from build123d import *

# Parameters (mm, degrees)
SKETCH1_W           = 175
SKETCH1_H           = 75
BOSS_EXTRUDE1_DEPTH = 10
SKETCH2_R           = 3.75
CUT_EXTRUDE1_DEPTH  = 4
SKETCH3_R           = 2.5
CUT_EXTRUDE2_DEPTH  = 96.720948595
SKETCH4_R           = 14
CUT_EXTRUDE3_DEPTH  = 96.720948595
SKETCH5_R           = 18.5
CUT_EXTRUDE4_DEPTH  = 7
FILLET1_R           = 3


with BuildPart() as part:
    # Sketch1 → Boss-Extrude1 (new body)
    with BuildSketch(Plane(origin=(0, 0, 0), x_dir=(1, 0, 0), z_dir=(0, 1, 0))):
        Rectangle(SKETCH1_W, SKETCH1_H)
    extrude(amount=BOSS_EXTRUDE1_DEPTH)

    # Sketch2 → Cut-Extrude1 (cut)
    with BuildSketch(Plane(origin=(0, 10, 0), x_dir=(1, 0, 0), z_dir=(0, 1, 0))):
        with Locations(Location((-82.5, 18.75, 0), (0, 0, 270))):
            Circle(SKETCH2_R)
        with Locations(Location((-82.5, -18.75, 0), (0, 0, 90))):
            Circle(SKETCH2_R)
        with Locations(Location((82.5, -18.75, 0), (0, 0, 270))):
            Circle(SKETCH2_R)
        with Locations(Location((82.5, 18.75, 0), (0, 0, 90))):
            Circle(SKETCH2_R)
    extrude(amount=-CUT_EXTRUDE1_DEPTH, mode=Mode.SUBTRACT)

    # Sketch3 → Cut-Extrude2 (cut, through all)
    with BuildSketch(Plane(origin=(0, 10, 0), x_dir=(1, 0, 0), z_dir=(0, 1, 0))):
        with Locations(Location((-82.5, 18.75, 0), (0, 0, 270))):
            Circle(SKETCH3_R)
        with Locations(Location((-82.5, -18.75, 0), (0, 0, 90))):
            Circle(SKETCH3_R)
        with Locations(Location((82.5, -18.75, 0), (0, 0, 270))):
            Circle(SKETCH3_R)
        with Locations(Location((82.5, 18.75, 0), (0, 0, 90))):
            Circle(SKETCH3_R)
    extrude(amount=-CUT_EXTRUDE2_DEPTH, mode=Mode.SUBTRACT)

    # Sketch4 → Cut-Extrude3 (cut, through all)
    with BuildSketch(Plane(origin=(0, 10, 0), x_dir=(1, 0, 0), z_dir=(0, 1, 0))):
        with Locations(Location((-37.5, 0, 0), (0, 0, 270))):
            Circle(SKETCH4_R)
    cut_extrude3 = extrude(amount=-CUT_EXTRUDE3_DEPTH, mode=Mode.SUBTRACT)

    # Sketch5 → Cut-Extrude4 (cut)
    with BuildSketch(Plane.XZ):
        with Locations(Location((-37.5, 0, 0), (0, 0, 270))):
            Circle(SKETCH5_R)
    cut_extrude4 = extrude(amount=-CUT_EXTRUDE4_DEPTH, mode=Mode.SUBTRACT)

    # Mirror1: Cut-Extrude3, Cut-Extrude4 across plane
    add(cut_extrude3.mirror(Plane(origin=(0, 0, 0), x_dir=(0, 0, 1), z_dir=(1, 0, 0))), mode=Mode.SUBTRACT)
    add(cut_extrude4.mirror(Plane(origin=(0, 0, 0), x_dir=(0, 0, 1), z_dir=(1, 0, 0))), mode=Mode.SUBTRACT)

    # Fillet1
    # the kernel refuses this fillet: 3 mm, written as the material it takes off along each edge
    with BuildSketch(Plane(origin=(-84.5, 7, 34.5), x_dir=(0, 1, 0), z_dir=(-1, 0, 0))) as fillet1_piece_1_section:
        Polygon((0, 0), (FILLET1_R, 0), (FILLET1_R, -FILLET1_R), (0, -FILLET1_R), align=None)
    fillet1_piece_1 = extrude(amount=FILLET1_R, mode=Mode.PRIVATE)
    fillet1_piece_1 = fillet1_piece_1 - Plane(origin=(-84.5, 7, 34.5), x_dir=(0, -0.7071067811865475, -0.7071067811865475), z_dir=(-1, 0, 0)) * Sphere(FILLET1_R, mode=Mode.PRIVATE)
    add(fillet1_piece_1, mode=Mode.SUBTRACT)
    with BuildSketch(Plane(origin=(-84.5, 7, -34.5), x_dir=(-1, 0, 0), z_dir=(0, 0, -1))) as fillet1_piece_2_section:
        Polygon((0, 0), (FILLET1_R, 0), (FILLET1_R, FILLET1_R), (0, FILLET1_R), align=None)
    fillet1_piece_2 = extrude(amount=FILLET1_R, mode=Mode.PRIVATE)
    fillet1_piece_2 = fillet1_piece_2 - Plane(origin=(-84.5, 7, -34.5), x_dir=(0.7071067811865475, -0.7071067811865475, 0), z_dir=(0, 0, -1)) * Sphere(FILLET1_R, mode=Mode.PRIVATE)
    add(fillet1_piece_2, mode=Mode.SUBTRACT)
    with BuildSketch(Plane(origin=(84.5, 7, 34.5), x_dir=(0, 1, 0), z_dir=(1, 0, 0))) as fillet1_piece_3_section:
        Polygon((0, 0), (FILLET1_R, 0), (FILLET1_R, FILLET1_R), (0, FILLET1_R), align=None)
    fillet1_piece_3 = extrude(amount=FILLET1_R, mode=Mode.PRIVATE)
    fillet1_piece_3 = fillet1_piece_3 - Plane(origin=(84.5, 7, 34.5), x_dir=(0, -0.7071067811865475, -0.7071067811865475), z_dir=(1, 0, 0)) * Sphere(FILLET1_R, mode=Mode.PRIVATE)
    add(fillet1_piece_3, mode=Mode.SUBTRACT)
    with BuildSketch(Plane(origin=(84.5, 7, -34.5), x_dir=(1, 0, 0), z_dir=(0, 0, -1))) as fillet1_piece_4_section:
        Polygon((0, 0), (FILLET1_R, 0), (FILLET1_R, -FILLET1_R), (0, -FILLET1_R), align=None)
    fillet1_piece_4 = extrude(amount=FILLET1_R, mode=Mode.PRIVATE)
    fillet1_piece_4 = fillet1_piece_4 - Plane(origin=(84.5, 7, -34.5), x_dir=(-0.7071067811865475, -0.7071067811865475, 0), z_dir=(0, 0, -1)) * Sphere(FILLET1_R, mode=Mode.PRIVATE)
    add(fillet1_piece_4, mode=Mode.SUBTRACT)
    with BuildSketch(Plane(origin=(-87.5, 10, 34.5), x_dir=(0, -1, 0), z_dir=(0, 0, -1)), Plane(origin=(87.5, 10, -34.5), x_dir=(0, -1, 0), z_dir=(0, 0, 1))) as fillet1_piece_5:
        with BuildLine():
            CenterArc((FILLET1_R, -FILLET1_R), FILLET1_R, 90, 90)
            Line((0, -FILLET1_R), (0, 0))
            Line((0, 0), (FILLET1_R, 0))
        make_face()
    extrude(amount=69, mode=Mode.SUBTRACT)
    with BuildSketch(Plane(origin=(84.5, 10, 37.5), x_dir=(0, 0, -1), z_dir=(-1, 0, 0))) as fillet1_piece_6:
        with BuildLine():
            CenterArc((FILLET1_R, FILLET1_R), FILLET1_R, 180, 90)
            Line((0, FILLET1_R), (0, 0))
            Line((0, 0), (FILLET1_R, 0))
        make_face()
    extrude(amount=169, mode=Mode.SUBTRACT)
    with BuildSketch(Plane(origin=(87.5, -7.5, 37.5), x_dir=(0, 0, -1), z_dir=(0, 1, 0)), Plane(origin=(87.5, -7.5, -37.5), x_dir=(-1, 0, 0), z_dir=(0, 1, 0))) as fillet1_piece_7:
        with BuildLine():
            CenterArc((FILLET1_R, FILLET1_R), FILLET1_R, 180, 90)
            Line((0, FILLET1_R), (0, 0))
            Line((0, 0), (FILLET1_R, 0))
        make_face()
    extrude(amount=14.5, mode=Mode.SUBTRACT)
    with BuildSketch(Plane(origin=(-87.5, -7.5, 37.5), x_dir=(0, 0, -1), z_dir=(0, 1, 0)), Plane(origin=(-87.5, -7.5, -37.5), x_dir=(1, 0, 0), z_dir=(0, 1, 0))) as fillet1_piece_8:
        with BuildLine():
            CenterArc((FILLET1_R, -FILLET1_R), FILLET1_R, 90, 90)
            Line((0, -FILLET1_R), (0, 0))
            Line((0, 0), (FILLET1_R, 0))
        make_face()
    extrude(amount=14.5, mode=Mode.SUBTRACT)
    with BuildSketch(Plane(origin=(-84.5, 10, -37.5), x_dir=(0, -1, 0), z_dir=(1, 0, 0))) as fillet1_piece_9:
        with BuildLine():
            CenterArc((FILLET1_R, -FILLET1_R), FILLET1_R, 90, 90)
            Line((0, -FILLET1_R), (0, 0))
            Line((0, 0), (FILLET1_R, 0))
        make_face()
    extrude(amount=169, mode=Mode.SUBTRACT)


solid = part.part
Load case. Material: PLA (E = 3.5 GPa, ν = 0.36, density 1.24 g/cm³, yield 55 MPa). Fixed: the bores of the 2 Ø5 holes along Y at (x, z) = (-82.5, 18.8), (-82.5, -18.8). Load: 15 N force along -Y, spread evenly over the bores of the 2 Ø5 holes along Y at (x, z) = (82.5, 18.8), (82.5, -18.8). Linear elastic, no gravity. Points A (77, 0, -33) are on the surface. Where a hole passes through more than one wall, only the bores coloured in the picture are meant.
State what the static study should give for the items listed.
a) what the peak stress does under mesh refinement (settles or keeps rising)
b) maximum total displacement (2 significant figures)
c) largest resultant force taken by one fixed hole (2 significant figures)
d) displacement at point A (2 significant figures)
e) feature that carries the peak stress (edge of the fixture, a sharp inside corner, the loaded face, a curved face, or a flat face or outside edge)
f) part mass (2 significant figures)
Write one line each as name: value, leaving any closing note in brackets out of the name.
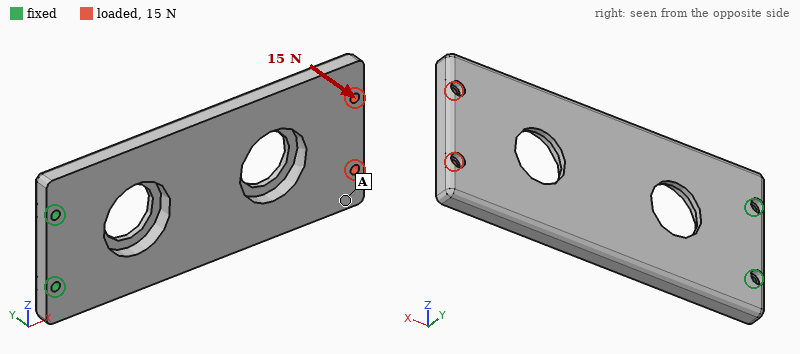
what the peak stress does under mesh refinement: keeps rising
maximum total displacement: 1.8 mm
largest resultant force taken by one fixed hole: 7.8 N
displacement at point A: 1.7 mm
feature that carries the peak stress: edge of the fixture
part mass: 140 g
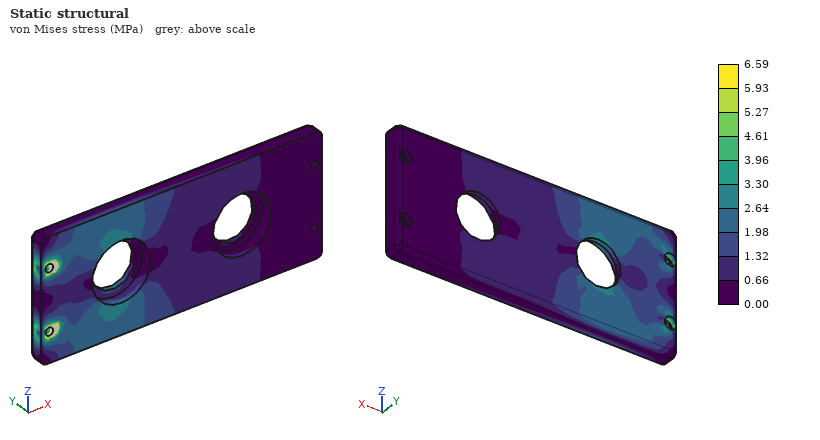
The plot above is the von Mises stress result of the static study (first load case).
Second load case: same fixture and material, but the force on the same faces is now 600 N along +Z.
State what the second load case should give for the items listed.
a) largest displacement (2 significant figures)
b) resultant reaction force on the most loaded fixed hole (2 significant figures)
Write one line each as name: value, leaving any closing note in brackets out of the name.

largest displacement: 2.1 mm
resultant reaction force on the most loaded fixed hole: 2.5 kN
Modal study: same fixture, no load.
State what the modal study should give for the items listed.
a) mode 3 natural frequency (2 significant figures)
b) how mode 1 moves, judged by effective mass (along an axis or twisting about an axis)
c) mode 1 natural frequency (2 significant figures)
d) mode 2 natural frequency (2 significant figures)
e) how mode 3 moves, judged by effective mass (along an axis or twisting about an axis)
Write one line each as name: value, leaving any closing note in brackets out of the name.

mode 3 natural frequency: 440 Hz
how mode 1 moves, judged by effective mass: along Y
mode 1 natural frequency: 75 Hz
mode 2 natural frequency: 350 Hz
how mode 3 moves, judged by effective mass: along Z
